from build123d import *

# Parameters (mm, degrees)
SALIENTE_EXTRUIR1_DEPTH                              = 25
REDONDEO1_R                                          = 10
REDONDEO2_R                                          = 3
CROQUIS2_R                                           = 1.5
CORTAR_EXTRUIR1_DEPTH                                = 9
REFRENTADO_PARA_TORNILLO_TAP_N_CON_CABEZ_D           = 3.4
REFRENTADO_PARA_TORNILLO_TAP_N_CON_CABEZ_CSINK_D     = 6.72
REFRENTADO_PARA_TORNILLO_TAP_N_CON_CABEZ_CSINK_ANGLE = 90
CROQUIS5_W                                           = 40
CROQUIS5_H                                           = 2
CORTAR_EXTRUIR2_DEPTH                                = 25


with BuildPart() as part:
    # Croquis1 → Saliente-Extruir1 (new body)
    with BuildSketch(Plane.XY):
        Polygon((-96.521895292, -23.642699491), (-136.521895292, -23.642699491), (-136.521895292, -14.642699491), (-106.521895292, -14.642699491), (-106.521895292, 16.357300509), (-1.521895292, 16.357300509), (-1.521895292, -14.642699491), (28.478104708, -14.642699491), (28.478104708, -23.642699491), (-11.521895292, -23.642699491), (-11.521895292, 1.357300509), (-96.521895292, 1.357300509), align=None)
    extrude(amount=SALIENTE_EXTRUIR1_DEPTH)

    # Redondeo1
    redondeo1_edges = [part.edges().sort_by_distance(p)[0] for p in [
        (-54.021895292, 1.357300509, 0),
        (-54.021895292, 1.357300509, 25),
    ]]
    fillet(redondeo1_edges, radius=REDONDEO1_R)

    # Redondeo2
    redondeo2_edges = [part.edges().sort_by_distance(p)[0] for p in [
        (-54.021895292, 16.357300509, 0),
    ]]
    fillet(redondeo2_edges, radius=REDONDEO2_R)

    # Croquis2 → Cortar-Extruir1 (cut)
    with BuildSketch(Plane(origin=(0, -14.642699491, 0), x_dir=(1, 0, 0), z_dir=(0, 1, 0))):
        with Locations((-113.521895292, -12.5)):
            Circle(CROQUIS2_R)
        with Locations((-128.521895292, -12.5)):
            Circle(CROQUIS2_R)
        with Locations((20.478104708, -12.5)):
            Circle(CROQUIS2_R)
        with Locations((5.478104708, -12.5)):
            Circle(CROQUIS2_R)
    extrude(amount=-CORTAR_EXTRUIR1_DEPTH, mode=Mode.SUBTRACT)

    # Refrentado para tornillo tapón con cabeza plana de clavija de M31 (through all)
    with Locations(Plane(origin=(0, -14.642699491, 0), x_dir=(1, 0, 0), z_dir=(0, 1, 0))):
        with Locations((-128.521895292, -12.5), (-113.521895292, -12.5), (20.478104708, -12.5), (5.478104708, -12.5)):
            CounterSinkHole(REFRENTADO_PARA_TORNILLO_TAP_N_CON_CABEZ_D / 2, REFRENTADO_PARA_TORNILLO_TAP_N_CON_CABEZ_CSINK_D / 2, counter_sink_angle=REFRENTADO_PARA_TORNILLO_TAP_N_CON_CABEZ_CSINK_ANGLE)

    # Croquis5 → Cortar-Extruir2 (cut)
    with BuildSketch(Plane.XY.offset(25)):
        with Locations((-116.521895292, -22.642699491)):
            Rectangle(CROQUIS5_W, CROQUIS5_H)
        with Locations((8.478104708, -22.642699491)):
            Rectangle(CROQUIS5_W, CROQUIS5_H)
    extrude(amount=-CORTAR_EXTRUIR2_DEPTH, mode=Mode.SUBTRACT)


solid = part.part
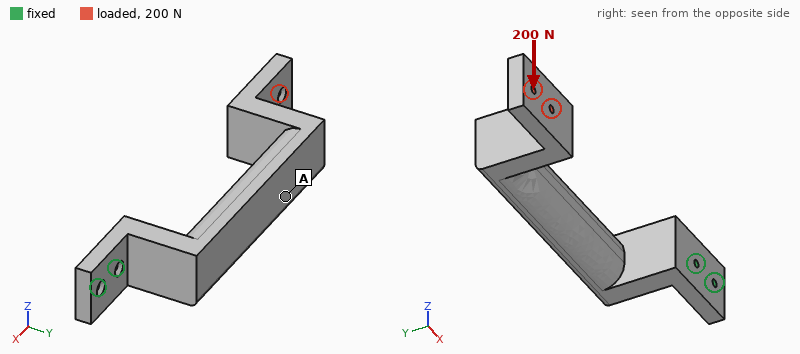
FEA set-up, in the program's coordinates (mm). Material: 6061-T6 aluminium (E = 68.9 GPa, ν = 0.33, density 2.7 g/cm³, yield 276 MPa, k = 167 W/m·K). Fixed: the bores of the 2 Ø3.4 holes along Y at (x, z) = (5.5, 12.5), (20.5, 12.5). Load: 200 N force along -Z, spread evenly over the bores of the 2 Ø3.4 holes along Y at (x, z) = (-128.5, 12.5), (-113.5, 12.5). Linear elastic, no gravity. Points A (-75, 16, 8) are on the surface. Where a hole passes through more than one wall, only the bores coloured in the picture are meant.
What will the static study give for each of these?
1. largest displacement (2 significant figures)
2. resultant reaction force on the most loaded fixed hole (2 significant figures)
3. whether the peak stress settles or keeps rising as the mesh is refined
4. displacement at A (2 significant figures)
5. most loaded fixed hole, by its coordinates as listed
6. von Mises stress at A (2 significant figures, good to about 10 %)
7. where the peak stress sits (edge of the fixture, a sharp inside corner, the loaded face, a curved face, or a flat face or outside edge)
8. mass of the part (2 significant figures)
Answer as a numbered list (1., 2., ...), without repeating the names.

1. 0.70 mm
2. 1.6 kN
3. keeps rising
4. 0.29 mm
5. (5.5, 12.5)
6. 6.9 MPa
7. edge of the fixture
8. 150 g
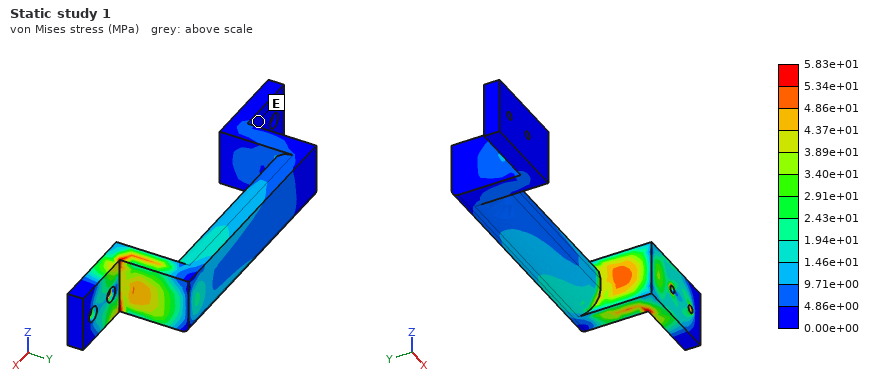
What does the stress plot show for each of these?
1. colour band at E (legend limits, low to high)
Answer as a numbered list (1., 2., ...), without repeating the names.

1. 0.00e+00 to 4.86e+00 MPa
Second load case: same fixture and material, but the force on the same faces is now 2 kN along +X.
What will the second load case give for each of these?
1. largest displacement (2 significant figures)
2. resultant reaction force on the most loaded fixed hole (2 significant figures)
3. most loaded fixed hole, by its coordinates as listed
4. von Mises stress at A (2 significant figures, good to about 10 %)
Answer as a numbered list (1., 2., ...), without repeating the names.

1. 2.0 mm
2. 1.5 kN
3. (5.5, 12.5)
4. 66 MPa
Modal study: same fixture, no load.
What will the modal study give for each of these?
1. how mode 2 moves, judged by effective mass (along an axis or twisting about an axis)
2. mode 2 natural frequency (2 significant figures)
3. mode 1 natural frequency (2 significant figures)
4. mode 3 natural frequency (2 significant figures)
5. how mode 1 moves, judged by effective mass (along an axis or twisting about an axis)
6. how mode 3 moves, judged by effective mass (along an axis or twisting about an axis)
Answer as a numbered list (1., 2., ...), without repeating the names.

1. along Z
2. 440 Hz
3. 260 Hz
4. 1300 Hz
5. along Y
6. along Z
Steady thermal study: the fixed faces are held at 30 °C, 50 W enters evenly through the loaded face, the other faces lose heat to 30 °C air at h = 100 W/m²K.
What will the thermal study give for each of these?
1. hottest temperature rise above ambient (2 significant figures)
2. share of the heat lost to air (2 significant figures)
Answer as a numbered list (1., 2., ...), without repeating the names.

1. 80 K
2. 81 %
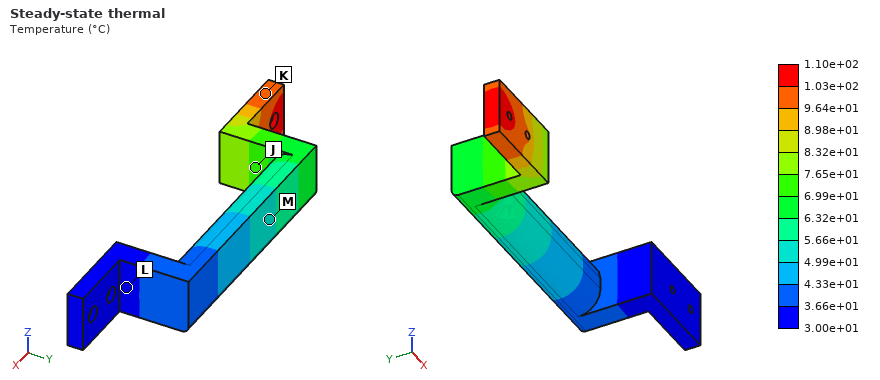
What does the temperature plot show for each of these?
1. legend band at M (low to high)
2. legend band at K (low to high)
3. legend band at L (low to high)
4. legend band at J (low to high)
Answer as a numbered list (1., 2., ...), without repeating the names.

1. 4.99e+01 to 5.66e+01 °C
2. 9.64e+01 to 1.03e+02 °C
3. 3.00e+01 to 3.66e+01 °C
4. 6.99e+01 to 7.65e+01 °C
